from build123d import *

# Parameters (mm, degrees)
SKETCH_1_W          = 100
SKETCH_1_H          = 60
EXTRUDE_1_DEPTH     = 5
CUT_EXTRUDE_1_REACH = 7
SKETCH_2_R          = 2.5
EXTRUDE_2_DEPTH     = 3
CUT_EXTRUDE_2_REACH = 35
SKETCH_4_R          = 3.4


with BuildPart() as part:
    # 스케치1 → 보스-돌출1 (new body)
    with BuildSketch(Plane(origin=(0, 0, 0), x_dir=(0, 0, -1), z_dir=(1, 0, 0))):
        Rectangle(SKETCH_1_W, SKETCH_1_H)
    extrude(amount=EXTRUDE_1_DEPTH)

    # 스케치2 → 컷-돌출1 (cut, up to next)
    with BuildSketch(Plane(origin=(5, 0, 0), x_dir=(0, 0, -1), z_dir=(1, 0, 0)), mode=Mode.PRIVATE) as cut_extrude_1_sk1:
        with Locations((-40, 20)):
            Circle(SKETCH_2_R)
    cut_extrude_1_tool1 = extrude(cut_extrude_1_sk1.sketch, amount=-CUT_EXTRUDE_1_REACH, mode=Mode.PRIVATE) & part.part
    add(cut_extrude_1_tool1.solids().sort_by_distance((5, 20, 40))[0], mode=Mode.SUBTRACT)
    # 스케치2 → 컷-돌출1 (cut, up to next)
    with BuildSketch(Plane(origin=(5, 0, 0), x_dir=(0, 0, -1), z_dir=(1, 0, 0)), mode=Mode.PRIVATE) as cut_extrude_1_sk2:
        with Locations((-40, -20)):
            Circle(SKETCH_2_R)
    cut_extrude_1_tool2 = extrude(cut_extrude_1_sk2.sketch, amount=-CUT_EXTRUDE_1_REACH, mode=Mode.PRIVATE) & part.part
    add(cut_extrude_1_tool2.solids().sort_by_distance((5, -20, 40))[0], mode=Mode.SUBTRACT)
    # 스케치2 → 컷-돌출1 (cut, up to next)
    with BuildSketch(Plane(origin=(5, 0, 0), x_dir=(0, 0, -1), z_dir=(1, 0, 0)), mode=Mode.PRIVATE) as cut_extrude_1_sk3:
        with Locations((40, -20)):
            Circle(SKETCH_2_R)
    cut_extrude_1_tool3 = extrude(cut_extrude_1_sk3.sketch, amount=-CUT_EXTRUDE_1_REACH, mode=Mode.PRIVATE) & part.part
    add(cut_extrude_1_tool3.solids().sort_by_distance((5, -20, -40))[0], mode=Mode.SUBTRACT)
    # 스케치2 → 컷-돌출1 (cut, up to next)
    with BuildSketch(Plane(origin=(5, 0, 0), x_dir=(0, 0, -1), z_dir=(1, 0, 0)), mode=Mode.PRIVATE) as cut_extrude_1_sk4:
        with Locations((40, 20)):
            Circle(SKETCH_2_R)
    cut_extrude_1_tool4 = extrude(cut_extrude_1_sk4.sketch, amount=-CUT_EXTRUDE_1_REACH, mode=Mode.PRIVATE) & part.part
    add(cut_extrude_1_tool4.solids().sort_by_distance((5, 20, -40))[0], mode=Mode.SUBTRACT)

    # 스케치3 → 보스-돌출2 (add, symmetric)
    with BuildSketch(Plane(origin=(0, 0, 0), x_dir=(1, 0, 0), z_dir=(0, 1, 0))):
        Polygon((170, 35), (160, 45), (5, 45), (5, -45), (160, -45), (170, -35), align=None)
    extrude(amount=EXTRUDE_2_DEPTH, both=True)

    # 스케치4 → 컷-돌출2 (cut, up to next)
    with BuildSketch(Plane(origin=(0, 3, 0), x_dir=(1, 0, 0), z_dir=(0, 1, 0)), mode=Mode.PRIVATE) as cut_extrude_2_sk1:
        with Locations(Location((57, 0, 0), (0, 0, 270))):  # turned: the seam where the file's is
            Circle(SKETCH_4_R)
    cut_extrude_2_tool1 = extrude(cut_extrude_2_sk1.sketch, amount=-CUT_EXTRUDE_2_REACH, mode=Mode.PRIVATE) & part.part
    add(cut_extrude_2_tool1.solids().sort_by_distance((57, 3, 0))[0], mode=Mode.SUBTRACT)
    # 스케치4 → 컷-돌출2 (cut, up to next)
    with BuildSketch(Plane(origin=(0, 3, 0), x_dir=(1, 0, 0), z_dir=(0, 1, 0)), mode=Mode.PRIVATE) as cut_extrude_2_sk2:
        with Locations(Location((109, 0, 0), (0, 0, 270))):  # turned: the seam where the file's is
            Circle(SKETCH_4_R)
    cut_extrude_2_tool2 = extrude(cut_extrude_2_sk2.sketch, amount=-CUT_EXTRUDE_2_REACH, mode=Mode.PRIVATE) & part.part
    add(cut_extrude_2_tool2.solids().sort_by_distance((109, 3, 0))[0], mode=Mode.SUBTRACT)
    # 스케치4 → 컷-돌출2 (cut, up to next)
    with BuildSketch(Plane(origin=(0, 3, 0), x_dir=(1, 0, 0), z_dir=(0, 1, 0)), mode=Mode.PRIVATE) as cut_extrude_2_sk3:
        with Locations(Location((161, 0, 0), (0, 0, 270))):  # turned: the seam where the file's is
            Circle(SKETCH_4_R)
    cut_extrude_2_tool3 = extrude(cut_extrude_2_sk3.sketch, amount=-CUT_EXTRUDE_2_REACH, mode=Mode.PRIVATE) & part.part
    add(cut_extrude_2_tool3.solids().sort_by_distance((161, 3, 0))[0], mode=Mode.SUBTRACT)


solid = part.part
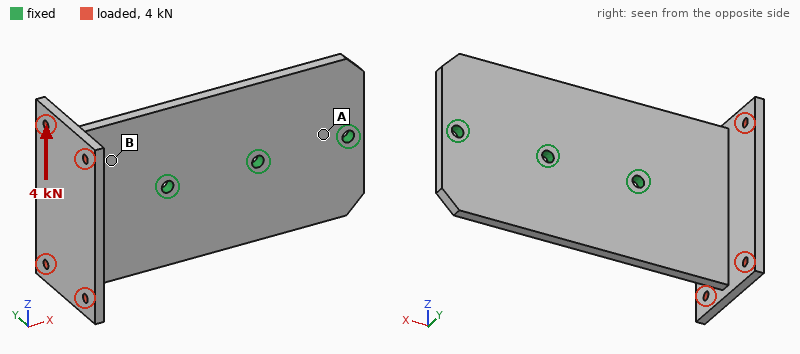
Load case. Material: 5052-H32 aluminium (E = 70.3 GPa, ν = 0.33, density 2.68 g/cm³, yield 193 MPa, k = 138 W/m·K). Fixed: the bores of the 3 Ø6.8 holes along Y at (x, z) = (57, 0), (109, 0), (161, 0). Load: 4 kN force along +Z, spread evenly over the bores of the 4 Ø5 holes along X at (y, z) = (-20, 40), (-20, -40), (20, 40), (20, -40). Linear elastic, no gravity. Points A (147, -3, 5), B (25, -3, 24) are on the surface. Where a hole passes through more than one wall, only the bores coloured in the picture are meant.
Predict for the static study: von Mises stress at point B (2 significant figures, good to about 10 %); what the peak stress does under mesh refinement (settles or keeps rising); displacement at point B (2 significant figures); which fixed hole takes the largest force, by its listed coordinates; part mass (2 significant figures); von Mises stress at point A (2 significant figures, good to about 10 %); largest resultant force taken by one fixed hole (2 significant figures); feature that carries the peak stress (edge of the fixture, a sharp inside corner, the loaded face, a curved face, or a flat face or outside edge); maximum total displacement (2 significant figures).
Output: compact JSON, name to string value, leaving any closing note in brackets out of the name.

{"von Mises stress at point B": "15 MPa", "what the peak stress does under mesh refinement": "keeps rising", "displacement at point B": "37 µm", "which fixed hole takes the largest force, by its listed coordinates": "(57, 0)", "part mass": "310 g", "von Mises stress at point A": "6.6 MPa", "largest resultant force taken by one fixed hole": "6.5 kN", "feature that carries the peak stress": "edge of the fixture", "maximum total displacement": "74 µm"}
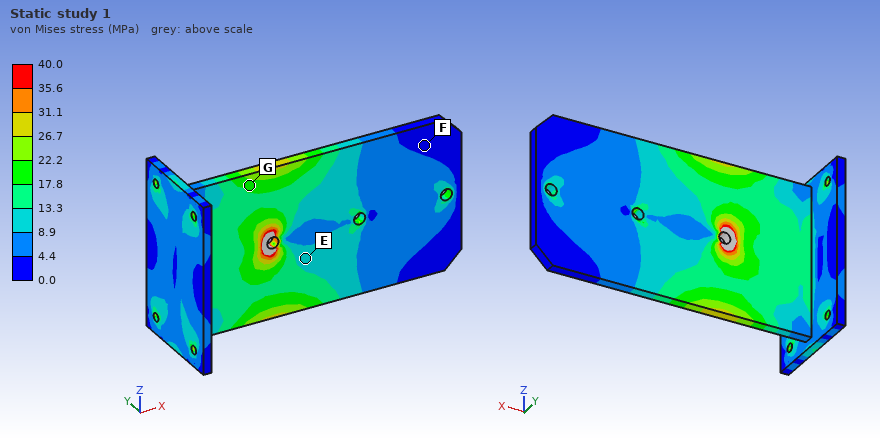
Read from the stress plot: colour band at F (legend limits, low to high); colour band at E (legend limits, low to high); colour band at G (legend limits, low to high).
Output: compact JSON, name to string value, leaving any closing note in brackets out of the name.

{"colour band at F": "0.0 to 4.4 MPa", "colour band at E": "8.9 to 13.3 MPa", "colour band at G": "17.8 to 22.2 MPa"}
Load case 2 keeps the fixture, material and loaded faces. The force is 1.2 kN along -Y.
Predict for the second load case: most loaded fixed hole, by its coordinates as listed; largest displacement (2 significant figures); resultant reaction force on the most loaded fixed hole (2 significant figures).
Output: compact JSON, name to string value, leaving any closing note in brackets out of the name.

{"most loaded fixed hole, by its coordinates as listed": "(57, 0)", "largest displacement": "0.91 mm", "resultant reaction force on the most loaded fixed hole": "1.8 kN"}
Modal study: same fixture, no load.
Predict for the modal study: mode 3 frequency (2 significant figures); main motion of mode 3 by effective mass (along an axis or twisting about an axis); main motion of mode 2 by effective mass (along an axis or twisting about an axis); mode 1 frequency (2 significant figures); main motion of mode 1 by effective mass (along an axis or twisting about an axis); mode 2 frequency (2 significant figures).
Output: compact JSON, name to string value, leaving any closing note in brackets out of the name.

{"mode 3 frequency": "2200 Hz", "main motion of mode 3 by effective mass": "twisting about X", "main motion of mode 2 by effective mass": "twisting about X", "mode 1 frequency": "620 Hz", "main motion of mode 1 by effective mass": "along Y", "mode 2 frequency": "840 Hz"}
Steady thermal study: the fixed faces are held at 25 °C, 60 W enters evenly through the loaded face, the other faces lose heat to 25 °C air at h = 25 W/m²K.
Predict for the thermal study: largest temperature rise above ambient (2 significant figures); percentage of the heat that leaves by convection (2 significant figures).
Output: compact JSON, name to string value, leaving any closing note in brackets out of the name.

{"largest temperature rise above ambient": "55 K", "percentage of the heat that leaves by convection": "36 %"}
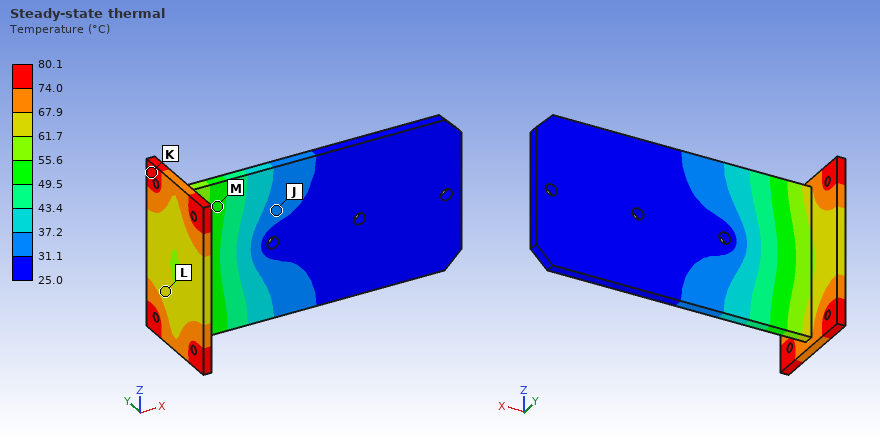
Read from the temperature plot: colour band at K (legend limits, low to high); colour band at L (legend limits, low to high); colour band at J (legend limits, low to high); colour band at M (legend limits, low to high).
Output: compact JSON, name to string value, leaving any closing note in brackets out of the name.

{"colour band at K": "74.0 to 80.1 °C", "colour band at L": "61.7 to 67.9 °C", "colour band at J": "31.1 to 37.2 °C", "colour band at M": "49.5 to 55.6 °C"}
